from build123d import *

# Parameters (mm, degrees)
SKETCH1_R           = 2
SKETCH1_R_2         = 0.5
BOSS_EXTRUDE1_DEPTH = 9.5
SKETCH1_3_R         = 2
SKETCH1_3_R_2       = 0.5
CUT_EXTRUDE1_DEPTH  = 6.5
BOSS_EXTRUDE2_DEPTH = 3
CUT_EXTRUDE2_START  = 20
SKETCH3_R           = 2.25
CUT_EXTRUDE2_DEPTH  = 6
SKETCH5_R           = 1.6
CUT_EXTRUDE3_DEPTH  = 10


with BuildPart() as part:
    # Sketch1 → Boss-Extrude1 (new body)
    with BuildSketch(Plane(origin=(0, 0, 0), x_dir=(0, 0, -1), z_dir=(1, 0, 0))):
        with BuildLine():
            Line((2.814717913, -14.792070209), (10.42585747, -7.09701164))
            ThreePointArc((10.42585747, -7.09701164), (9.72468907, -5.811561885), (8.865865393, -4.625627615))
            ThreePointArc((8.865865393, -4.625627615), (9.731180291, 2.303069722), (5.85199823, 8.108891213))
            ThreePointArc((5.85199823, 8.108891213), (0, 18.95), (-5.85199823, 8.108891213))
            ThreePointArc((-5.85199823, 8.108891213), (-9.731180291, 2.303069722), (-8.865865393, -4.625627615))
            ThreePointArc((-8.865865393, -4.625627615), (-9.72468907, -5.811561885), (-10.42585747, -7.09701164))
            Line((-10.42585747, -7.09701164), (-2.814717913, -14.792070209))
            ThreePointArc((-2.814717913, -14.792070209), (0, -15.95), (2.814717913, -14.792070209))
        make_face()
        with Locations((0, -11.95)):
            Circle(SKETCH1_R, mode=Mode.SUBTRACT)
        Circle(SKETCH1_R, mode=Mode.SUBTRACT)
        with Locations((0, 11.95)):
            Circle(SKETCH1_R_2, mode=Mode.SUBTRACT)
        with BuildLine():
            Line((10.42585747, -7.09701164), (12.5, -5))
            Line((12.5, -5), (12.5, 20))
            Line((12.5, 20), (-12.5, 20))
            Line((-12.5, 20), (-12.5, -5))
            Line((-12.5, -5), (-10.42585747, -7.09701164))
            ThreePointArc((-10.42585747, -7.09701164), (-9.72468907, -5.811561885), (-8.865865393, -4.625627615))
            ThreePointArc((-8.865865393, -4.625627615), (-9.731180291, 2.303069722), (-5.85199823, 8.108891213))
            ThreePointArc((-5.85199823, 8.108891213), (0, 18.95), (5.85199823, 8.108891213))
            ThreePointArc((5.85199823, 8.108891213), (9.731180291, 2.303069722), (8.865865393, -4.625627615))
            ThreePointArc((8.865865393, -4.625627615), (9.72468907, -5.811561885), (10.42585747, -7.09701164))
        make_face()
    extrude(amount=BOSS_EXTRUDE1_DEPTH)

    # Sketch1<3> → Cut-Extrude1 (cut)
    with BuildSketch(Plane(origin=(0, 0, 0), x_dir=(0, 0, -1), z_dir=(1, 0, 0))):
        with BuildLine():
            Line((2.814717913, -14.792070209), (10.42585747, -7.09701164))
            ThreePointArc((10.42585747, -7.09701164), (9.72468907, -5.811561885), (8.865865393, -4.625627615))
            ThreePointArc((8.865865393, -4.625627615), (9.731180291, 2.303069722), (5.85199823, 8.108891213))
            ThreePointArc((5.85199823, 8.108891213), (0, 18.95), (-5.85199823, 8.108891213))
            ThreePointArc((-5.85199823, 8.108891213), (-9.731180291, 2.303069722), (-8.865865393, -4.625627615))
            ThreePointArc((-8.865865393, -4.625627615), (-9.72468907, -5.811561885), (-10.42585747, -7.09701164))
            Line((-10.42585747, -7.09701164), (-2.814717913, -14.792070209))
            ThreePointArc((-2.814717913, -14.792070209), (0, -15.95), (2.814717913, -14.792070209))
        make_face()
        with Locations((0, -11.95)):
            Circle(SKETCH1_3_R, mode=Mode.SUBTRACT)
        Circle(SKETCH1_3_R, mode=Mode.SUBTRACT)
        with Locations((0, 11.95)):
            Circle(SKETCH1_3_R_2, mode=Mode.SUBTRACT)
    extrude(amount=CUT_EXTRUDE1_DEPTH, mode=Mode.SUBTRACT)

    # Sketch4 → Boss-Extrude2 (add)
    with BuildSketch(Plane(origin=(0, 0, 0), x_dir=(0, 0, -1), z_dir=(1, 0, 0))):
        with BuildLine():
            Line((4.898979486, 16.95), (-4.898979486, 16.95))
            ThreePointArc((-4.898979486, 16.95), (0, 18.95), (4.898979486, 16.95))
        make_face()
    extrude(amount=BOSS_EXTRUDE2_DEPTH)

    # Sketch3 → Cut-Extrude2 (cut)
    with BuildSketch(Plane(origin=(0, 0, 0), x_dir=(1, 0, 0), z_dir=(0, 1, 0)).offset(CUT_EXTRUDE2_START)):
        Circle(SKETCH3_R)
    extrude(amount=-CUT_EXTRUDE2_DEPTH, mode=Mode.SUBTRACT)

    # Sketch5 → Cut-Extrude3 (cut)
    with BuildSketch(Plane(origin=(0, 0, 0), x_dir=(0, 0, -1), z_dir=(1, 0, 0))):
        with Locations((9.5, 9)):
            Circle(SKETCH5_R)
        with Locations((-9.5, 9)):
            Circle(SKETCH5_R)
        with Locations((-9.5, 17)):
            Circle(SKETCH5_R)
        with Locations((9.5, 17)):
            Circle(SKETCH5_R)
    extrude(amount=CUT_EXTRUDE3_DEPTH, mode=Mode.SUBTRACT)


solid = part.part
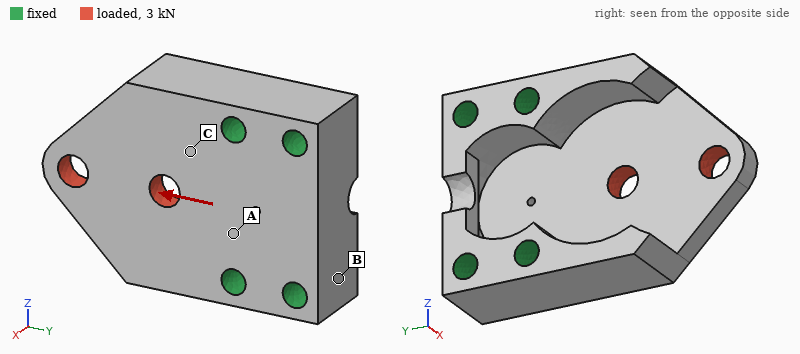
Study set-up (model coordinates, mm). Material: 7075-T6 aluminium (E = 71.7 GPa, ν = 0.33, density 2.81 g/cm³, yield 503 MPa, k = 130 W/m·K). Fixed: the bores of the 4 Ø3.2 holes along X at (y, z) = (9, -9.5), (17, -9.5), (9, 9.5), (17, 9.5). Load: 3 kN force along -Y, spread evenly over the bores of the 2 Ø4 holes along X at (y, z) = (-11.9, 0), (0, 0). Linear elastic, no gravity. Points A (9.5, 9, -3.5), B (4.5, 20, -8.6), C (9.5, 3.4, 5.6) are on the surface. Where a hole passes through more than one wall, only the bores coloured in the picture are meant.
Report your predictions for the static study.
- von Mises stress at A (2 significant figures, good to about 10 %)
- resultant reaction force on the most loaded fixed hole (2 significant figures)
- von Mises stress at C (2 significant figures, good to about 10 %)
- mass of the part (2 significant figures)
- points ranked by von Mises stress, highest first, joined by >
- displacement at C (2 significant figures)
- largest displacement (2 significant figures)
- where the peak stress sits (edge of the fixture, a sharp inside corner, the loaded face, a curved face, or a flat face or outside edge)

30 MPa
1.3 kN
55 MPa
10 g
C > A > B
5.5 µm
23 µm
the loaded face
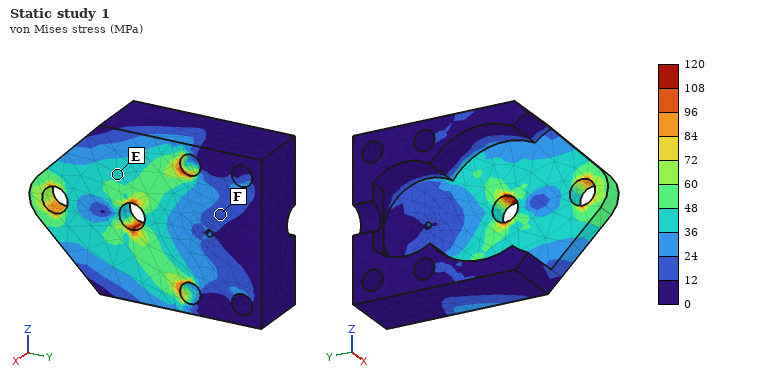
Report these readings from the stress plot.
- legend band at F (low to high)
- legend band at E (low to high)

12 to 24 MPa
36 to 48 MPa
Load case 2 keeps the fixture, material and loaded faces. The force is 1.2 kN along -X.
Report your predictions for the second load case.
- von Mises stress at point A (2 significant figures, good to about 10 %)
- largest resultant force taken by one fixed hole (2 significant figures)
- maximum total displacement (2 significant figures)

69 MPa
730 N
0.25 mm
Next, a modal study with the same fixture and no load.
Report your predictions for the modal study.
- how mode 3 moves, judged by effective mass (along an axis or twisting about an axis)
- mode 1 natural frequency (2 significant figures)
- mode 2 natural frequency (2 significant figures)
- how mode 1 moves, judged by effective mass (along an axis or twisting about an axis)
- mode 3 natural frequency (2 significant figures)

along Z
12 kHz
25 kHz
along X
30 kHz
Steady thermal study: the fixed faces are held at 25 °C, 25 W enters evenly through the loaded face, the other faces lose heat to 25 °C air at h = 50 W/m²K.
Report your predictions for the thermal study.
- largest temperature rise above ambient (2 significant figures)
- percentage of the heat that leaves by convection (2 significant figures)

48 K
5.0 %
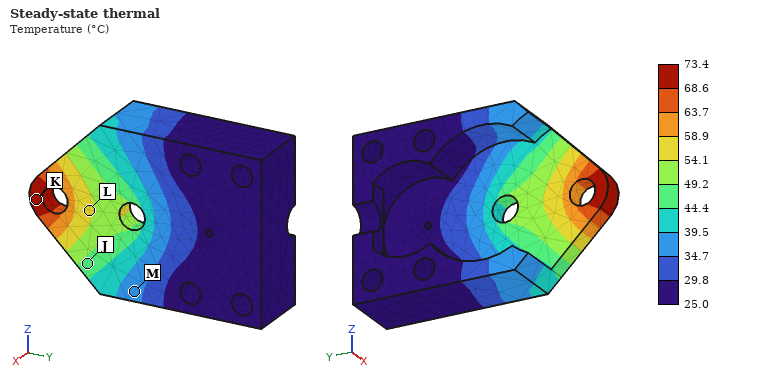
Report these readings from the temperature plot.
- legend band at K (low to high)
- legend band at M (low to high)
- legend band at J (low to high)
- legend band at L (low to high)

68.6 to 73.4 °C
34.7 to 39.5 °C
44.4 to 49.2 °C
54.1 to 58.9 °C
